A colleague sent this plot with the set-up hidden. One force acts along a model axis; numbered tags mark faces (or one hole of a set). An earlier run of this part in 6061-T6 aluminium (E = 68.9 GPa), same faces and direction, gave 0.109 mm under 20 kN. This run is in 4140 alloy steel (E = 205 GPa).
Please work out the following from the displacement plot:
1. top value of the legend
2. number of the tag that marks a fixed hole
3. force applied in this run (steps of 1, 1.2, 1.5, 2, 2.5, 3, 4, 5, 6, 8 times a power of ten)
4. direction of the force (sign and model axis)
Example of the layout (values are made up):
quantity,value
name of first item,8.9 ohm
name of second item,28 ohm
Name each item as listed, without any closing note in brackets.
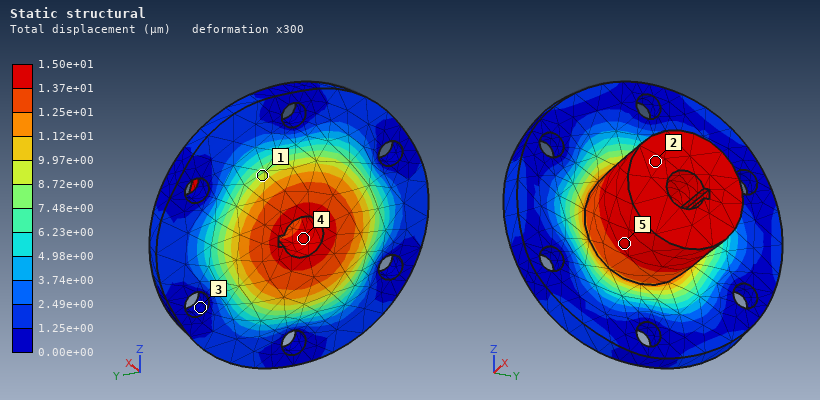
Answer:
quantity,value
top value of the legend,1.50e+01 µm
number of the tag that marks a fixed hole,3
force applied in this run,8 kN
direction of the force,-X
